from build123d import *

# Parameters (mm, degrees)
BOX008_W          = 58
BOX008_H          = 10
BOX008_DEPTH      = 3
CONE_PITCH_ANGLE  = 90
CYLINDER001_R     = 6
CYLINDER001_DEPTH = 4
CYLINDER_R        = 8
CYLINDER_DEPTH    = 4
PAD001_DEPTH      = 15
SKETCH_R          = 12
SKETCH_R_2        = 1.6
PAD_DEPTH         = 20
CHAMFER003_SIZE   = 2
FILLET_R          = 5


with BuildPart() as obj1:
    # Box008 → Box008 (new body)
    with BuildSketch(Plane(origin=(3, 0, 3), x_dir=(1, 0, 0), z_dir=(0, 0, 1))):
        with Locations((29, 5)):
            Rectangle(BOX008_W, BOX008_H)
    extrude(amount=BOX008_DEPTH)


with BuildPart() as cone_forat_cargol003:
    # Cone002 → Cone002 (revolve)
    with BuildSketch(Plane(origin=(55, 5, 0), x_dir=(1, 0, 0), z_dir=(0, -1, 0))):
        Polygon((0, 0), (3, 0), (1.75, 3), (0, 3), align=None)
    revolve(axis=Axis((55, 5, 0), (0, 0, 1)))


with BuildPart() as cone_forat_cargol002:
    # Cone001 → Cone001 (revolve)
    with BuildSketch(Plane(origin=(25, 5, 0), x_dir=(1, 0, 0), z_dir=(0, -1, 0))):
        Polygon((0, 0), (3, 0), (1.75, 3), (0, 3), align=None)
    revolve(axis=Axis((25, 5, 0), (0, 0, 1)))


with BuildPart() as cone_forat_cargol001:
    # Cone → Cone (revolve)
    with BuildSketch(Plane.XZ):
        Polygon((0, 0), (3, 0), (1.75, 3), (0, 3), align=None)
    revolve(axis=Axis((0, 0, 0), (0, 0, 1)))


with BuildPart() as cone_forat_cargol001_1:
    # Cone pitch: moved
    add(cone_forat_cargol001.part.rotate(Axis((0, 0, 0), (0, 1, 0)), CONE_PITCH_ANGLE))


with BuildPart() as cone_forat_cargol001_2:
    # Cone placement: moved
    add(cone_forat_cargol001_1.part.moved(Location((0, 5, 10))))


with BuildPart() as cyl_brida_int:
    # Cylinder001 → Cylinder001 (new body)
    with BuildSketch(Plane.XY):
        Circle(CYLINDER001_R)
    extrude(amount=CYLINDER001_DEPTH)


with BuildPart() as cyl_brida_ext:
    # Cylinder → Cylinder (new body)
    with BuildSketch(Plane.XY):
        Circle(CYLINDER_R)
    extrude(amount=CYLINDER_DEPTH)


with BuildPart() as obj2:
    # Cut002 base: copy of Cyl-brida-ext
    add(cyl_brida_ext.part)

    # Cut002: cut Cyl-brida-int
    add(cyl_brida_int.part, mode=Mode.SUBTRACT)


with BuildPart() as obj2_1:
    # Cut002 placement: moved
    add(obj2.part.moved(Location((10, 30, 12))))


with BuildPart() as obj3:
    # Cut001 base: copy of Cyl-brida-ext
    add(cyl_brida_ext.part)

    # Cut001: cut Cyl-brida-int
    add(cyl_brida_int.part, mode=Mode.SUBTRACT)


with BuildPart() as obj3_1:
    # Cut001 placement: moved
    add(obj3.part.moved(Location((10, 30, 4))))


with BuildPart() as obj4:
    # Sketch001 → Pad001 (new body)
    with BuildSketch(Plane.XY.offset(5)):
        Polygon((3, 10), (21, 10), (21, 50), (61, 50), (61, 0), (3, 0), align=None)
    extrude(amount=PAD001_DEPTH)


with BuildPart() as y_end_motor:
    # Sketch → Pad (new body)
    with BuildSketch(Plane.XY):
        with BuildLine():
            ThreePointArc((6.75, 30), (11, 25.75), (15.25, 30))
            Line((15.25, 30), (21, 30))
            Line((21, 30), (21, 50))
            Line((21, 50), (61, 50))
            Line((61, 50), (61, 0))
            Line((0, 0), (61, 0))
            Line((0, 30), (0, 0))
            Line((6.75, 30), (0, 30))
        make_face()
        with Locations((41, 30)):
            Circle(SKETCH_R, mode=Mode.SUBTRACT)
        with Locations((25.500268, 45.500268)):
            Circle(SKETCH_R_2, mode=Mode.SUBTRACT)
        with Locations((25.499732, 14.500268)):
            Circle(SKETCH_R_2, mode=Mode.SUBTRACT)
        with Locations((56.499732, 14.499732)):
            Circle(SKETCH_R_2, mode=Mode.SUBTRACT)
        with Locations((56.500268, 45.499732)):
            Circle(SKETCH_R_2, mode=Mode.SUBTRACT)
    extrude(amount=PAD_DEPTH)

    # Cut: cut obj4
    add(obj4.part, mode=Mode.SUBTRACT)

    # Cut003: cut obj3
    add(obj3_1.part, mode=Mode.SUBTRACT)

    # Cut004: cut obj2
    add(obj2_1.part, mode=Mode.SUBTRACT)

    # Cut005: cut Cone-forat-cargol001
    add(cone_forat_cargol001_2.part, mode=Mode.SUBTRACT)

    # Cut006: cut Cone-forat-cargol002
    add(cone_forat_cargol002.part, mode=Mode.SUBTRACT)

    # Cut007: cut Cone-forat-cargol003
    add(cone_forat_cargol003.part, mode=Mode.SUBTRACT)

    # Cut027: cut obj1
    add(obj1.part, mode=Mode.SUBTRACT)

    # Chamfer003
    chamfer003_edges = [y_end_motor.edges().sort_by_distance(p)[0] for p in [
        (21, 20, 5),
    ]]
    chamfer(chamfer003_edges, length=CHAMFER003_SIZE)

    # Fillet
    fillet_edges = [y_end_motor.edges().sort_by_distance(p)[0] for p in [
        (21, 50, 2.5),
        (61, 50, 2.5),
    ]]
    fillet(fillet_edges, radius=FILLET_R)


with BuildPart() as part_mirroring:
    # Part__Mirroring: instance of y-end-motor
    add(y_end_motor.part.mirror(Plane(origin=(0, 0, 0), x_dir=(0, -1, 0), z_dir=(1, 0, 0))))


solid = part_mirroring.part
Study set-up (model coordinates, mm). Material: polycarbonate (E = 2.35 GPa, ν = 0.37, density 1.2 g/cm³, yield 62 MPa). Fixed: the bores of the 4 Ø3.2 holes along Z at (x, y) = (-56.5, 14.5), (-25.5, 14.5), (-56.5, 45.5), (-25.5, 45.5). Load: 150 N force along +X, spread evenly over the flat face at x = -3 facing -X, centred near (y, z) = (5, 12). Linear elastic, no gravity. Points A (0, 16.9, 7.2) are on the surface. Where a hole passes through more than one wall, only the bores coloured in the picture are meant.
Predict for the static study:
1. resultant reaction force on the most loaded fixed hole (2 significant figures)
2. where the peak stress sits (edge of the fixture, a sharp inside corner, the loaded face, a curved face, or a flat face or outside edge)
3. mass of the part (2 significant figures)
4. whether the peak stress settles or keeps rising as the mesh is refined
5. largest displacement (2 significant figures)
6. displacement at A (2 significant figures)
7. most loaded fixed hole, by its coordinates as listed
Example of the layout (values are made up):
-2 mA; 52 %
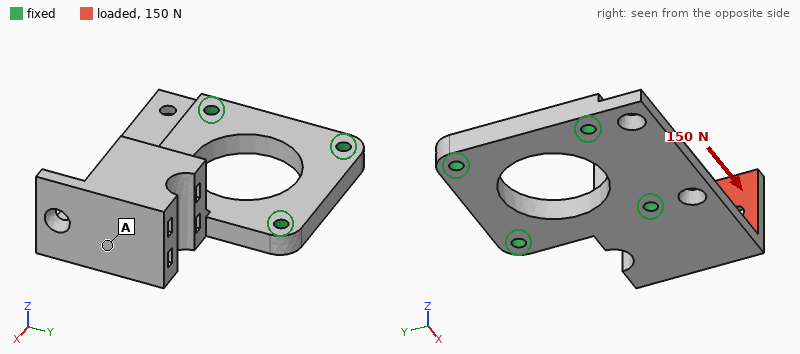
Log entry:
160 N; edge of the fixture; 18 g; keeps rising; 0.87 mm; 0.44 mm; (-25.5, 14.5)
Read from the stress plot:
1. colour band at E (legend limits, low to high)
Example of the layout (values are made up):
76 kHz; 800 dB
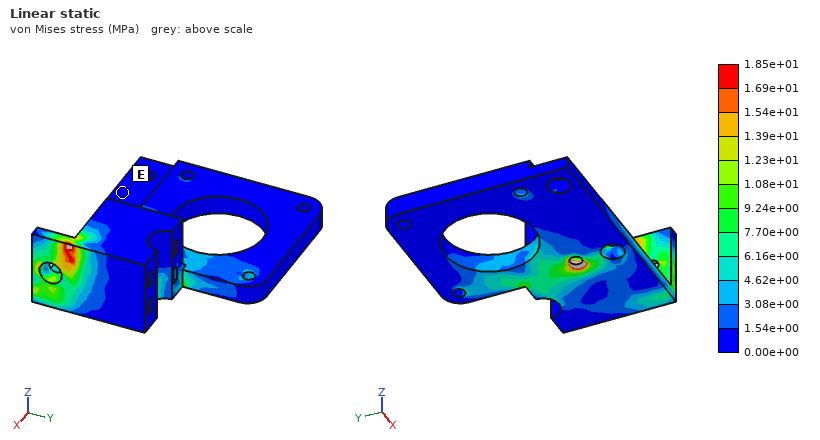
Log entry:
0.00e+00 to 1.54e+00 MPa
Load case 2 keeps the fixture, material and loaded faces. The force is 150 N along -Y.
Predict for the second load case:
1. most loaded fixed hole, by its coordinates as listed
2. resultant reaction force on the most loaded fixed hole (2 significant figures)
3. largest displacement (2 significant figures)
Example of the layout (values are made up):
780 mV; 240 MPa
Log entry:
(-25.5, 14.5); 130 N; 0.28 mm
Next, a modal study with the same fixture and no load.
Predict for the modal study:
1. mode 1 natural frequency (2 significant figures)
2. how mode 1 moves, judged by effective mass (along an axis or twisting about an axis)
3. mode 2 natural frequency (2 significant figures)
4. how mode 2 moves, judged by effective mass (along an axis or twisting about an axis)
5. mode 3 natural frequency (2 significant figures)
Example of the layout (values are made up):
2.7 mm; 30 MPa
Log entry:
790 Hz; along Z; 1700 Hz; along Y; 2700 Hz
